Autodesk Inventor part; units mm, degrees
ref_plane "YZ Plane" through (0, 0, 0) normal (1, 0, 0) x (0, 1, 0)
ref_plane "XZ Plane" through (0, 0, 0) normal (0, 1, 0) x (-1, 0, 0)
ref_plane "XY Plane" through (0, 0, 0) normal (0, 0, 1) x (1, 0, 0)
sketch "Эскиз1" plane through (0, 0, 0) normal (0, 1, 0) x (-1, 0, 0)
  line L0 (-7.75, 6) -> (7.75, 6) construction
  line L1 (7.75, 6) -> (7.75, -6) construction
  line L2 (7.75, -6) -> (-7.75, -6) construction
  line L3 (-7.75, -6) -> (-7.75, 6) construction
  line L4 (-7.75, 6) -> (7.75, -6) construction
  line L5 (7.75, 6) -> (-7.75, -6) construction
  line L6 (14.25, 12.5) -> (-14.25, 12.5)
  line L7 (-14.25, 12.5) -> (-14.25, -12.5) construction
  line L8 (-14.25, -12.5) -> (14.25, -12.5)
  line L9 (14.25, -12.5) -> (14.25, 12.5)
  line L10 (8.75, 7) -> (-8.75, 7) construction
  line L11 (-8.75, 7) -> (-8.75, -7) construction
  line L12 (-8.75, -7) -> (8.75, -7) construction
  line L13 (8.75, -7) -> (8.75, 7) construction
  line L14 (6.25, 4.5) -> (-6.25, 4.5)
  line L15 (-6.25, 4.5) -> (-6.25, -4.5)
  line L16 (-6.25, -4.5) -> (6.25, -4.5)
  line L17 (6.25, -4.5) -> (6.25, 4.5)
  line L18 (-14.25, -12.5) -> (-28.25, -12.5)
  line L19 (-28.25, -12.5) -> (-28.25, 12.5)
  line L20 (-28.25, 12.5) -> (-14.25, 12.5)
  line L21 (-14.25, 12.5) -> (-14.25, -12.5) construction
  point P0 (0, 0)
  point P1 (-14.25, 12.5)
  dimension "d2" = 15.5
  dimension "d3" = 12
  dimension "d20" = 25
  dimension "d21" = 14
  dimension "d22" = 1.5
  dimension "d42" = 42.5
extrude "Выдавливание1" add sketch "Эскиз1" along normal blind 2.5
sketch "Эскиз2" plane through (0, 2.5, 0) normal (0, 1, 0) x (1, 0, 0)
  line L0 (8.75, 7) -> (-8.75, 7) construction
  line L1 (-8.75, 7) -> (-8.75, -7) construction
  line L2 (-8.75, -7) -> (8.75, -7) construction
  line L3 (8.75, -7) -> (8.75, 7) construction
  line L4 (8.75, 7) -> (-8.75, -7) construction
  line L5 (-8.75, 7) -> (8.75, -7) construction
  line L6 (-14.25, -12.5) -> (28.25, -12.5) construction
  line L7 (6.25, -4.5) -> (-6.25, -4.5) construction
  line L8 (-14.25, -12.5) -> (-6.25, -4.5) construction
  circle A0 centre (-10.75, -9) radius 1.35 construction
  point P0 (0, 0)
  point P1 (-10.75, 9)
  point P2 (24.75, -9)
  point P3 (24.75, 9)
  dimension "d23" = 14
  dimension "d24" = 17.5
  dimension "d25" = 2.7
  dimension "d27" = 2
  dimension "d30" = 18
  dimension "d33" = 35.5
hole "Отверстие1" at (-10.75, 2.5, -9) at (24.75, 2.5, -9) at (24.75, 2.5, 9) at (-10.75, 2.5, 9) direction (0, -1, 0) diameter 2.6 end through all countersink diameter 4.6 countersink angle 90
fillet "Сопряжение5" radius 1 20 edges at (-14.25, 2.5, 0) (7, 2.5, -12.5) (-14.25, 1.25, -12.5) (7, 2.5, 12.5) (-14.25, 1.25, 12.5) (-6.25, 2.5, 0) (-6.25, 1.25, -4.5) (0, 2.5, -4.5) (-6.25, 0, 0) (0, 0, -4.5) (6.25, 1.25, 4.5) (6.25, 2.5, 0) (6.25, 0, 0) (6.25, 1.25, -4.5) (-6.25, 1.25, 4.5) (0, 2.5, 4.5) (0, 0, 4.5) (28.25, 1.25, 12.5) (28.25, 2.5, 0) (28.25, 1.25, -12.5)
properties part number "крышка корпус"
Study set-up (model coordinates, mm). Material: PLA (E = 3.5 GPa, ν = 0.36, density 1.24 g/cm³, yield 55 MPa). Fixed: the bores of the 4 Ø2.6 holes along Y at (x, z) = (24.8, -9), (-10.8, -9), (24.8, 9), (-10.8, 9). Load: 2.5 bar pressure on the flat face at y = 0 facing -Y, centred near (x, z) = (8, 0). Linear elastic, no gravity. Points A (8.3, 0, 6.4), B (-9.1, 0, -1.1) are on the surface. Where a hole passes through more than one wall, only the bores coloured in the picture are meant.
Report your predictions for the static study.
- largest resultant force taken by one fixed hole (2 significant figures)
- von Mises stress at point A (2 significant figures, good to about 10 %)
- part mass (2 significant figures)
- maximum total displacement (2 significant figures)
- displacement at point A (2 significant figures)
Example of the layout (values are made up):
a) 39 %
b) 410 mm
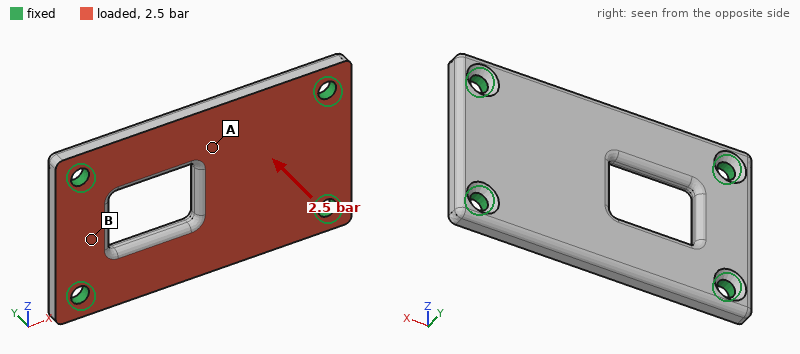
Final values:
a) 65 N
b) 12 MPa
c) 2.8 g
d) 0.33 mm
e) 0.29 mm
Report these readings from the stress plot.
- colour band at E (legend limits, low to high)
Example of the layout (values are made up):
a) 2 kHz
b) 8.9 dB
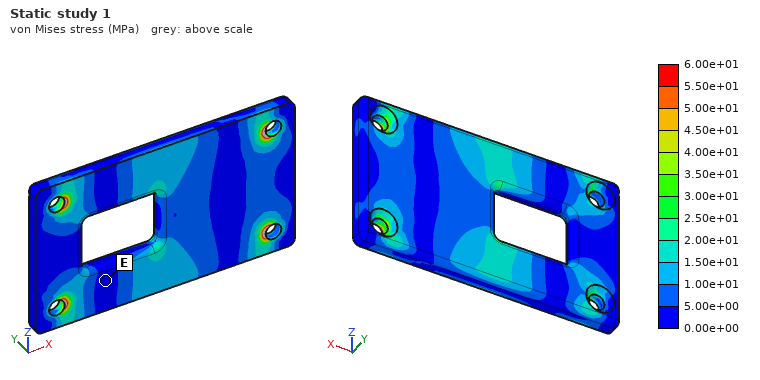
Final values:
a) 0.00e+00 to 5.00e+00 MPa
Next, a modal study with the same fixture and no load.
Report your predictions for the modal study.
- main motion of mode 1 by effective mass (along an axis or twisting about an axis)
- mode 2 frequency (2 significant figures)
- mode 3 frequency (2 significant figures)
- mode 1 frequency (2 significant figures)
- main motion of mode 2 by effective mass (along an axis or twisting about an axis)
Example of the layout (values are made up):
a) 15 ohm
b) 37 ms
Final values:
a) along Y
b) 4100 Hz
c) 7700 Hz
d) 2900 Hz
e) twisting about X
